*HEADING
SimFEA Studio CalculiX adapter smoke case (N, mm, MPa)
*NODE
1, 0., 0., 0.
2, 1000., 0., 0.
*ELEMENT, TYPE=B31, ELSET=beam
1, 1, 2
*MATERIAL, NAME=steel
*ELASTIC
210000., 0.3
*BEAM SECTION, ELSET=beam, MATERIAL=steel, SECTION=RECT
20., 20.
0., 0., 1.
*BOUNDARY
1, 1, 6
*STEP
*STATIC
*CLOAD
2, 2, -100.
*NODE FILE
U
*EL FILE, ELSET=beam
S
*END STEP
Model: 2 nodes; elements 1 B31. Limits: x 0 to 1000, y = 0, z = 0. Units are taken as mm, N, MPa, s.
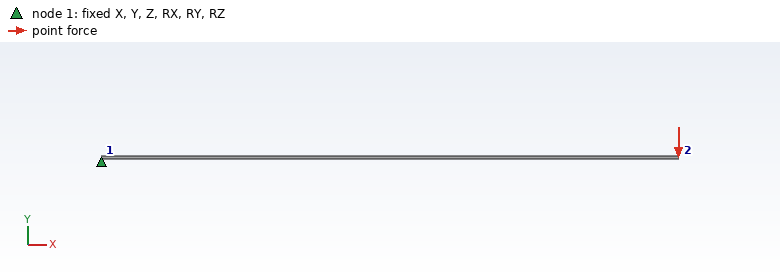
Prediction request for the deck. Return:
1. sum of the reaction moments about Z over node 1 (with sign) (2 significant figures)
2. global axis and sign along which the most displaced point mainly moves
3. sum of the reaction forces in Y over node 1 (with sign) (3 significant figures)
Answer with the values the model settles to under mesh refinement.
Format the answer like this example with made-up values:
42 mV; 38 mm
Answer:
100000 N·mm; -Y; 100 N
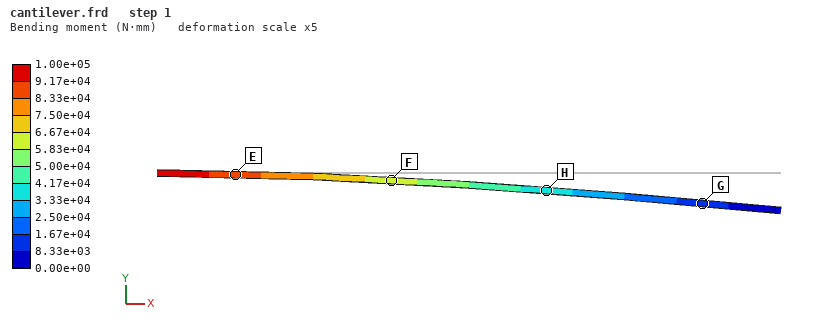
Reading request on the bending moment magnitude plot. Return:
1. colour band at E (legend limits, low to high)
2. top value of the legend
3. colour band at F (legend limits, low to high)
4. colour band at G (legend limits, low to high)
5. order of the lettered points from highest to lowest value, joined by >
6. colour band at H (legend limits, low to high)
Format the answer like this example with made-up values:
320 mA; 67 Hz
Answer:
8.33e+04 to 9.17e+04 N·mm; 1.00e+05 N·mm; 5.83e+04 to 6.67e+04 N·mm; 8.33e+03 to 1.67e+04 N·mm; E > F > H > G; 3.33e+04 to 4.17e+04 N·mm
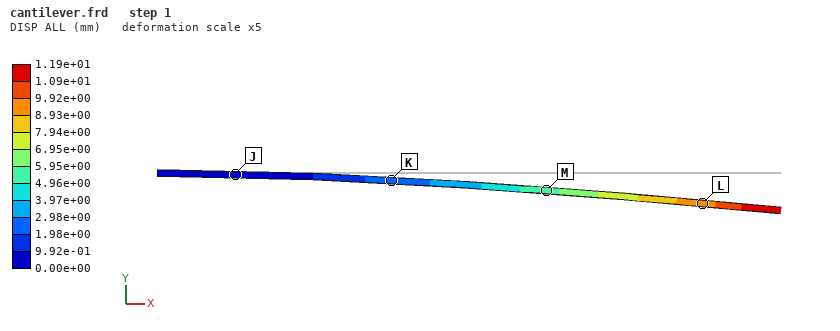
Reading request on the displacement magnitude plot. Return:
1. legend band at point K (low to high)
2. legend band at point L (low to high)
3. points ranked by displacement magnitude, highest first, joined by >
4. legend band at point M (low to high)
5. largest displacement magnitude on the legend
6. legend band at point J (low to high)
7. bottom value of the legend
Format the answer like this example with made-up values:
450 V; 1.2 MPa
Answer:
1.98e+00 to 2.98e+00 mm; 8.93e+00 to 9.92e+00 mm; L > M > K > J; 4.96e+00 to 5.95e+00 mm; 1.19e+01 mm; 0.00e+00 to 9.92e-01 mm; 0.00e+00 mm
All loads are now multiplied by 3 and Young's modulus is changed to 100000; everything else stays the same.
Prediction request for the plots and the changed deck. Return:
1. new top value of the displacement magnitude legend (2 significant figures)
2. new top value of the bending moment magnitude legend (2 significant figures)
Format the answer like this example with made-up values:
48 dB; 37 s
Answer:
75 mm; 3.0e+05 N·mm
